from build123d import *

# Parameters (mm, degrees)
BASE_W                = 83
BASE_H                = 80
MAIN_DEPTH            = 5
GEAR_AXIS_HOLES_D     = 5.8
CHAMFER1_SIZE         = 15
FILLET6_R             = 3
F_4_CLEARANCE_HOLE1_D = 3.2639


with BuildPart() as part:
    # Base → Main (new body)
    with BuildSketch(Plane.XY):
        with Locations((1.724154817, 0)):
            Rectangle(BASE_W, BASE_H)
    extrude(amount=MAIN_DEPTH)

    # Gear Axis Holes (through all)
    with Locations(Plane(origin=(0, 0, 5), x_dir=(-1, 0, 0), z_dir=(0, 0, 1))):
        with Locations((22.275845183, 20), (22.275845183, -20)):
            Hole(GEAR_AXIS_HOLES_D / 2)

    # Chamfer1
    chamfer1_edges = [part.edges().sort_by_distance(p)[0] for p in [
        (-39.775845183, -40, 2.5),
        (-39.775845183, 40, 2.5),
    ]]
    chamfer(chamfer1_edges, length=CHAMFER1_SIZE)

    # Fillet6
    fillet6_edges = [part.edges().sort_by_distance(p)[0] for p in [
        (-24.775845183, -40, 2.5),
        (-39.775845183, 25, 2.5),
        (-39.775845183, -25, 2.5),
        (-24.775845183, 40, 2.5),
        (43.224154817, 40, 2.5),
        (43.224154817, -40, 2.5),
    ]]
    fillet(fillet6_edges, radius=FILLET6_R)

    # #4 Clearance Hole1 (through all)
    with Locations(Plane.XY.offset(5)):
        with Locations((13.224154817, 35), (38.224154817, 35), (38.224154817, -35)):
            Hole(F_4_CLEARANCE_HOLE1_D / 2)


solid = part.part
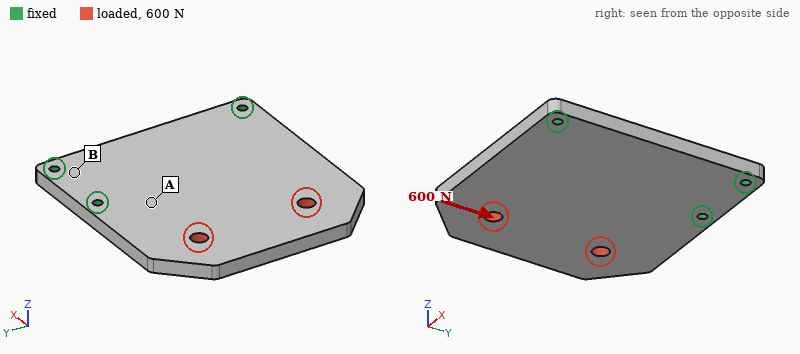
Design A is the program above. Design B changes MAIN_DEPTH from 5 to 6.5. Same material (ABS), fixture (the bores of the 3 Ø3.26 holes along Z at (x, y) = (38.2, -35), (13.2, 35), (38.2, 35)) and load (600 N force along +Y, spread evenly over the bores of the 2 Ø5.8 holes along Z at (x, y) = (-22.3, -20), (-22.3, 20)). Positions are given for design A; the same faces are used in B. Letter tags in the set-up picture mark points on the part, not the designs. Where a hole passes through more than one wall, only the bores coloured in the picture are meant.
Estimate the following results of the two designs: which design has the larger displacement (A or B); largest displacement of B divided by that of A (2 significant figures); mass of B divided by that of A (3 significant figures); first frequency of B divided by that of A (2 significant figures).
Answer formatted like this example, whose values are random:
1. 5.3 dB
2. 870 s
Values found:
1. A
2. 0.77
3. 1.30
4. 1.3
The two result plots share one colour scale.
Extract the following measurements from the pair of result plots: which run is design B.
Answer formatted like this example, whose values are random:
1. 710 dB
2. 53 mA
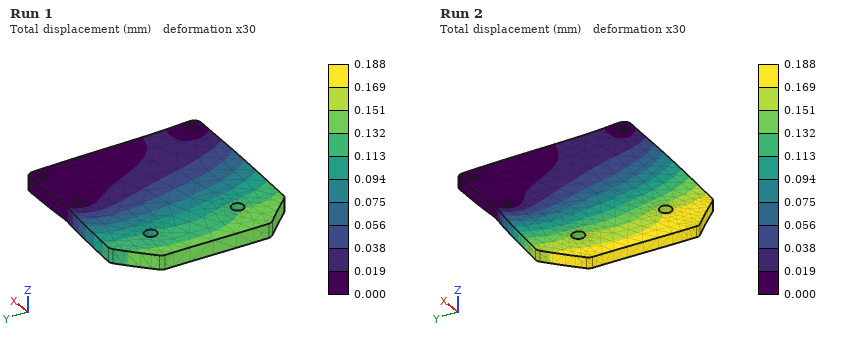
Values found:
1. Run 1
